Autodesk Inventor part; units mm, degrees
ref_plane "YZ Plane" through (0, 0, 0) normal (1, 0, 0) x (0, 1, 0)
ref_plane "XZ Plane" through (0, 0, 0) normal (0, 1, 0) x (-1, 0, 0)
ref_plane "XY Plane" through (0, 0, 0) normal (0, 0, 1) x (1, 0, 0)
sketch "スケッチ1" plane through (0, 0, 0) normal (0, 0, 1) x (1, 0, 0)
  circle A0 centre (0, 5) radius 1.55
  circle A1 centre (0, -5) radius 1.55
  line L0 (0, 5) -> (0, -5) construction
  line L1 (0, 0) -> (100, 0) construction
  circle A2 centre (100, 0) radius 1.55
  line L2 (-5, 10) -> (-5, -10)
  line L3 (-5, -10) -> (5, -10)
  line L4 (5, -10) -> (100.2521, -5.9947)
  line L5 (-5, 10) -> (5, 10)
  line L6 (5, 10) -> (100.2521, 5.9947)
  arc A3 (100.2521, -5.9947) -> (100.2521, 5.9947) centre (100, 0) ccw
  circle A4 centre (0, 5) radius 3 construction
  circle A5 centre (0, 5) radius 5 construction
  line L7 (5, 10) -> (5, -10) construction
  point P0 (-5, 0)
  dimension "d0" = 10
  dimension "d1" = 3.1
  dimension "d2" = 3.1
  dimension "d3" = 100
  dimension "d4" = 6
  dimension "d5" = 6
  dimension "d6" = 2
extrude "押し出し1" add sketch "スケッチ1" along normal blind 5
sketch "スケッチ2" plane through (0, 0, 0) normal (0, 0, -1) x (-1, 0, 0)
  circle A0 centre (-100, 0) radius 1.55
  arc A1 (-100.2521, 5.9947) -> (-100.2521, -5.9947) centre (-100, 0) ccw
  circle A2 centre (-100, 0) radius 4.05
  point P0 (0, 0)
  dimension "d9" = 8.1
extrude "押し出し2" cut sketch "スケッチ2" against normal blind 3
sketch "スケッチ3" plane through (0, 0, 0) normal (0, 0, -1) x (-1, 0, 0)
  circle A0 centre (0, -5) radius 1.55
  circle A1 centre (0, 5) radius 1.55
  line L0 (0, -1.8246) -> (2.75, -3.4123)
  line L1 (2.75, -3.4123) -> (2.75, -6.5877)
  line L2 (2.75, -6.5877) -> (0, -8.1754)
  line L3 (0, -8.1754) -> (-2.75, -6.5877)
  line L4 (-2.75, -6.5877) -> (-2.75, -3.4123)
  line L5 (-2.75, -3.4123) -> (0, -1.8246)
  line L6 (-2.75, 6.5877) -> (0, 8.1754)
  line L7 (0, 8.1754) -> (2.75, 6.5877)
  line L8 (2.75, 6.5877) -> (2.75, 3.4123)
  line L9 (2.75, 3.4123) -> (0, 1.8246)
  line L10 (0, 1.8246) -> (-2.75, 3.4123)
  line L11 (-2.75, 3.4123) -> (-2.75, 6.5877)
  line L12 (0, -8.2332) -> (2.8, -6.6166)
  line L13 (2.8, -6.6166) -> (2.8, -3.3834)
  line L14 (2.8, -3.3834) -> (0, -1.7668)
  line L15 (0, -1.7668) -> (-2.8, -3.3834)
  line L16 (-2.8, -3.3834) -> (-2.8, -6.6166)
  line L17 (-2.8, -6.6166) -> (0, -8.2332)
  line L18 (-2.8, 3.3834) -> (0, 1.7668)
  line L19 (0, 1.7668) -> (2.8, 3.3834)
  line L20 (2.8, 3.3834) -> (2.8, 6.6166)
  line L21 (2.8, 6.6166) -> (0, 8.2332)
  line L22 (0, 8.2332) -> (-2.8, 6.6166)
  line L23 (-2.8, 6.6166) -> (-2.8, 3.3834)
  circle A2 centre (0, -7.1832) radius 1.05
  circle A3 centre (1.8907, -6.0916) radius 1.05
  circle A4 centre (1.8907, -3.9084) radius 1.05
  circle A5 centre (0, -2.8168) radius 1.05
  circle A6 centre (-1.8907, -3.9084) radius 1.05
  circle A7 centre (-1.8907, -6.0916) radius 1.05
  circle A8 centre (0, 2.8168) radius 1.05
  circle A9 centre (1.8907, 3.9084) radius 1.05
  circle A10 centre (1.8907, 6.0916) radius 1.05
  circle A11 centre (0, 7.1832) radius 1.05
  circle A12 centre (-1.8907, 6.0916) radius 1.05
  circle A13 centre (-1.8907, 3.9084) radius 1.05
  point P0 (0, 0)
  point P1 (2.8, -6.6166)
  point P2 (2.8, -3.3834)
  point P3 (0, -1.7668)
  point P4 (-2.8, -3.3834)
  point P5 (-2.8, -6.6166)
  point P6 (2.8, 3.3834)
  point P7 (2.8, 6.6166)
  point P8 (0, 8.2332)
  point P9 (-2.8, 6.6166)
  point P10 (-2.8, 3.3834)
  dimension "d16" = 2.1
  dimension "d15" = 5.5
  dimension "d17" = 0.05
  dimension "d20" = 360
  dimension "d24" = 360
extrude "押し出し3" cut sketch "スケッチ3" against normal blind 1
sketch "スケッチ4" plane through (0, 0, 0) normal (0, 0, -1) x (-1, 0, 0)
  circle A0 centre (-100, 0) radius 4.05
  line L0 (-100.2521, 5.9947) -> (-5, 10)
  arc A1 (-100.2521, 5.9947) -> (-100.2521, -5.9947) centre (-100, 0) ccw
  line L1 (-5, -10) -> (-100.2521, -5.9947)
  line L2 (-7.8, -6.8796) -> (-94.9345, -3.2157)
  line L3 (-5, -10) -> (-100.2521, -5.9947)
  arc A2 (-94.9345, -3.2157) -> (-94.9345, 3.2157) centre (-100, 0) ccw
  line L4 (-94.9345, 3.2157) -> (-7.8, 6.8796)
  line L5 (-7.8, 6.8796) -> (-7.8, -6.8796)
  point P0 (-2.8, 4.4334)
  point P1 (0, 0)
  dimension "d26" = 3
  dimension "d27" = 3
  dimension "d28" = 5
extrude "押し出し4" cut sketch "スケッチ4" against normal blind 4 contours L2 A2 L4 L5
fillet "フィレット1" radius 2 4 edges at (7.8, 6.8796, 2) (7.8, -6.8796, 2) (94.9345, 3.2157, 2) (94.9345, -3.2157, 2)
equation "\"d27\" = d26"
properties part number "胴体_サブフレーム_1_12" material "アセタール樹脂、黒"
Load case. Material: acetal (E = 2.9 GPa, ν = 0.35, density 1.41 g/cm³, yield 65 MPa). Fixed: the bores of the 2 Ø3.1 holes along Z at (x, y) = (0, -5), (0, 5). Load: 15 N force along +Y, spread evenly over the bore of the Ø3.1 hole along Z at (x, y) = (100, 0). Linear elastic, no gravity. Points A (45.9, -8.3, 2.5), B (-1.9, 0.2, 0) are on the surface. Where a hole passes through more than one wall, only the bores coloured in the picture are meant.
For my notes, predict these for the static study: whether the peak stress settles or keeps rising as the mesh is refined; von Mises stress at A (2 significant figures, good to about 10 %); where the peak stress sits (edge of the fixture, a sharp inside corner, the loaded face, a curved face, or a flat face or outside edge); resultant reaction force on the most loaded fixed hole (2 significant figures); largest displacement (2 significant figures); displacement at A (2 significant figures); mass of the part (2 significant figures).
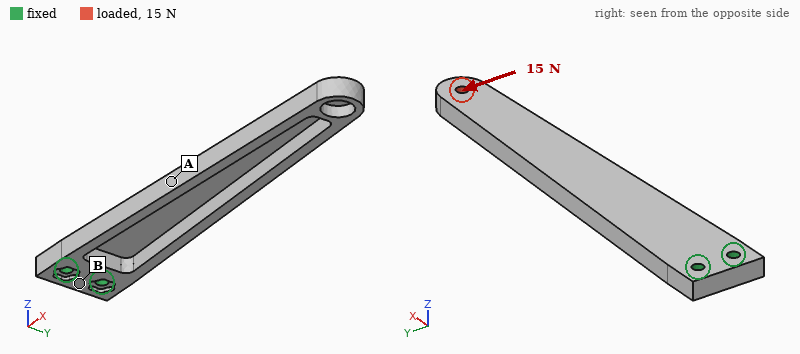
keeps rising
4.6 MPa
edge of the fixture
120 N
1.2 mm
0.28 mm
7.2 g
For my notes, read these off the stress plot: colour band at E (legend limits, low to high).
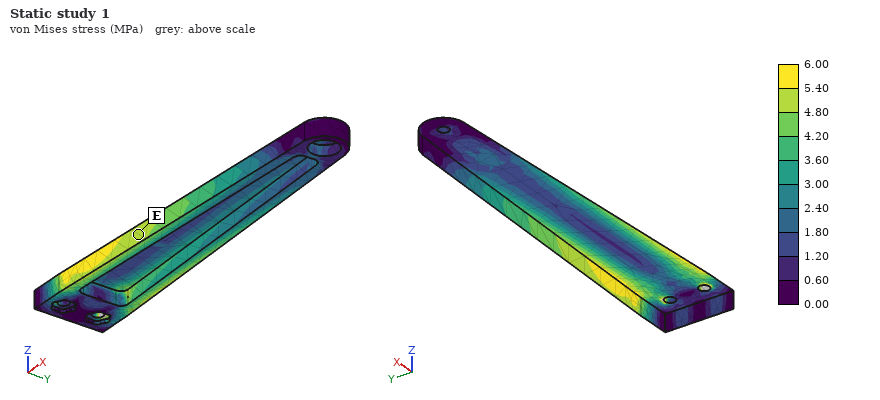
4.80 to 5.40 MPa
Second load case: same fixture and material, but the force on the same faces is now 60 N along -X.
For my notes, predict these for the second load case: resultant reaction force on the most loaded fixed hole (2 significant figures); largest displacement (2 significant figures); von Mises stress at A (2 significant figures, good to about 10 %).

30 N
1.1 mm
1.2 MPa
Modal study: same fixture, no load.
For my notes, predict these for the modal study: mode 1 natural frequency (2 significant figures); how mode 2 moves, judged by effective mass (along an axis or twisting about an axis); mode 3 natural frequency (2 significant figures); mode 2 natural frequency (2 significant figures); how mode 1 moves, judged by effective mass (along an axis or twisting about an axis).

120 Hz
along Y
680 Hz
430 Hz
along Z
